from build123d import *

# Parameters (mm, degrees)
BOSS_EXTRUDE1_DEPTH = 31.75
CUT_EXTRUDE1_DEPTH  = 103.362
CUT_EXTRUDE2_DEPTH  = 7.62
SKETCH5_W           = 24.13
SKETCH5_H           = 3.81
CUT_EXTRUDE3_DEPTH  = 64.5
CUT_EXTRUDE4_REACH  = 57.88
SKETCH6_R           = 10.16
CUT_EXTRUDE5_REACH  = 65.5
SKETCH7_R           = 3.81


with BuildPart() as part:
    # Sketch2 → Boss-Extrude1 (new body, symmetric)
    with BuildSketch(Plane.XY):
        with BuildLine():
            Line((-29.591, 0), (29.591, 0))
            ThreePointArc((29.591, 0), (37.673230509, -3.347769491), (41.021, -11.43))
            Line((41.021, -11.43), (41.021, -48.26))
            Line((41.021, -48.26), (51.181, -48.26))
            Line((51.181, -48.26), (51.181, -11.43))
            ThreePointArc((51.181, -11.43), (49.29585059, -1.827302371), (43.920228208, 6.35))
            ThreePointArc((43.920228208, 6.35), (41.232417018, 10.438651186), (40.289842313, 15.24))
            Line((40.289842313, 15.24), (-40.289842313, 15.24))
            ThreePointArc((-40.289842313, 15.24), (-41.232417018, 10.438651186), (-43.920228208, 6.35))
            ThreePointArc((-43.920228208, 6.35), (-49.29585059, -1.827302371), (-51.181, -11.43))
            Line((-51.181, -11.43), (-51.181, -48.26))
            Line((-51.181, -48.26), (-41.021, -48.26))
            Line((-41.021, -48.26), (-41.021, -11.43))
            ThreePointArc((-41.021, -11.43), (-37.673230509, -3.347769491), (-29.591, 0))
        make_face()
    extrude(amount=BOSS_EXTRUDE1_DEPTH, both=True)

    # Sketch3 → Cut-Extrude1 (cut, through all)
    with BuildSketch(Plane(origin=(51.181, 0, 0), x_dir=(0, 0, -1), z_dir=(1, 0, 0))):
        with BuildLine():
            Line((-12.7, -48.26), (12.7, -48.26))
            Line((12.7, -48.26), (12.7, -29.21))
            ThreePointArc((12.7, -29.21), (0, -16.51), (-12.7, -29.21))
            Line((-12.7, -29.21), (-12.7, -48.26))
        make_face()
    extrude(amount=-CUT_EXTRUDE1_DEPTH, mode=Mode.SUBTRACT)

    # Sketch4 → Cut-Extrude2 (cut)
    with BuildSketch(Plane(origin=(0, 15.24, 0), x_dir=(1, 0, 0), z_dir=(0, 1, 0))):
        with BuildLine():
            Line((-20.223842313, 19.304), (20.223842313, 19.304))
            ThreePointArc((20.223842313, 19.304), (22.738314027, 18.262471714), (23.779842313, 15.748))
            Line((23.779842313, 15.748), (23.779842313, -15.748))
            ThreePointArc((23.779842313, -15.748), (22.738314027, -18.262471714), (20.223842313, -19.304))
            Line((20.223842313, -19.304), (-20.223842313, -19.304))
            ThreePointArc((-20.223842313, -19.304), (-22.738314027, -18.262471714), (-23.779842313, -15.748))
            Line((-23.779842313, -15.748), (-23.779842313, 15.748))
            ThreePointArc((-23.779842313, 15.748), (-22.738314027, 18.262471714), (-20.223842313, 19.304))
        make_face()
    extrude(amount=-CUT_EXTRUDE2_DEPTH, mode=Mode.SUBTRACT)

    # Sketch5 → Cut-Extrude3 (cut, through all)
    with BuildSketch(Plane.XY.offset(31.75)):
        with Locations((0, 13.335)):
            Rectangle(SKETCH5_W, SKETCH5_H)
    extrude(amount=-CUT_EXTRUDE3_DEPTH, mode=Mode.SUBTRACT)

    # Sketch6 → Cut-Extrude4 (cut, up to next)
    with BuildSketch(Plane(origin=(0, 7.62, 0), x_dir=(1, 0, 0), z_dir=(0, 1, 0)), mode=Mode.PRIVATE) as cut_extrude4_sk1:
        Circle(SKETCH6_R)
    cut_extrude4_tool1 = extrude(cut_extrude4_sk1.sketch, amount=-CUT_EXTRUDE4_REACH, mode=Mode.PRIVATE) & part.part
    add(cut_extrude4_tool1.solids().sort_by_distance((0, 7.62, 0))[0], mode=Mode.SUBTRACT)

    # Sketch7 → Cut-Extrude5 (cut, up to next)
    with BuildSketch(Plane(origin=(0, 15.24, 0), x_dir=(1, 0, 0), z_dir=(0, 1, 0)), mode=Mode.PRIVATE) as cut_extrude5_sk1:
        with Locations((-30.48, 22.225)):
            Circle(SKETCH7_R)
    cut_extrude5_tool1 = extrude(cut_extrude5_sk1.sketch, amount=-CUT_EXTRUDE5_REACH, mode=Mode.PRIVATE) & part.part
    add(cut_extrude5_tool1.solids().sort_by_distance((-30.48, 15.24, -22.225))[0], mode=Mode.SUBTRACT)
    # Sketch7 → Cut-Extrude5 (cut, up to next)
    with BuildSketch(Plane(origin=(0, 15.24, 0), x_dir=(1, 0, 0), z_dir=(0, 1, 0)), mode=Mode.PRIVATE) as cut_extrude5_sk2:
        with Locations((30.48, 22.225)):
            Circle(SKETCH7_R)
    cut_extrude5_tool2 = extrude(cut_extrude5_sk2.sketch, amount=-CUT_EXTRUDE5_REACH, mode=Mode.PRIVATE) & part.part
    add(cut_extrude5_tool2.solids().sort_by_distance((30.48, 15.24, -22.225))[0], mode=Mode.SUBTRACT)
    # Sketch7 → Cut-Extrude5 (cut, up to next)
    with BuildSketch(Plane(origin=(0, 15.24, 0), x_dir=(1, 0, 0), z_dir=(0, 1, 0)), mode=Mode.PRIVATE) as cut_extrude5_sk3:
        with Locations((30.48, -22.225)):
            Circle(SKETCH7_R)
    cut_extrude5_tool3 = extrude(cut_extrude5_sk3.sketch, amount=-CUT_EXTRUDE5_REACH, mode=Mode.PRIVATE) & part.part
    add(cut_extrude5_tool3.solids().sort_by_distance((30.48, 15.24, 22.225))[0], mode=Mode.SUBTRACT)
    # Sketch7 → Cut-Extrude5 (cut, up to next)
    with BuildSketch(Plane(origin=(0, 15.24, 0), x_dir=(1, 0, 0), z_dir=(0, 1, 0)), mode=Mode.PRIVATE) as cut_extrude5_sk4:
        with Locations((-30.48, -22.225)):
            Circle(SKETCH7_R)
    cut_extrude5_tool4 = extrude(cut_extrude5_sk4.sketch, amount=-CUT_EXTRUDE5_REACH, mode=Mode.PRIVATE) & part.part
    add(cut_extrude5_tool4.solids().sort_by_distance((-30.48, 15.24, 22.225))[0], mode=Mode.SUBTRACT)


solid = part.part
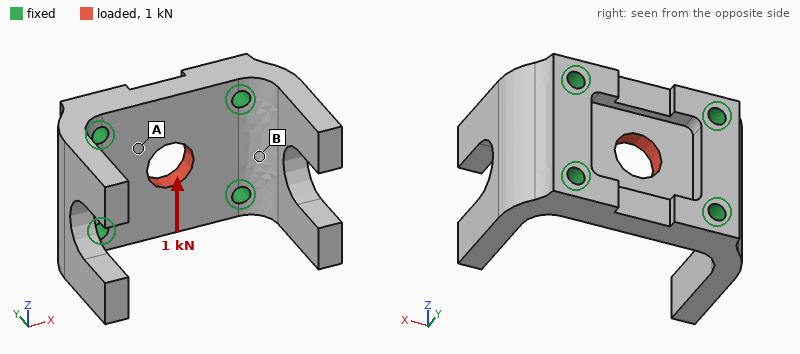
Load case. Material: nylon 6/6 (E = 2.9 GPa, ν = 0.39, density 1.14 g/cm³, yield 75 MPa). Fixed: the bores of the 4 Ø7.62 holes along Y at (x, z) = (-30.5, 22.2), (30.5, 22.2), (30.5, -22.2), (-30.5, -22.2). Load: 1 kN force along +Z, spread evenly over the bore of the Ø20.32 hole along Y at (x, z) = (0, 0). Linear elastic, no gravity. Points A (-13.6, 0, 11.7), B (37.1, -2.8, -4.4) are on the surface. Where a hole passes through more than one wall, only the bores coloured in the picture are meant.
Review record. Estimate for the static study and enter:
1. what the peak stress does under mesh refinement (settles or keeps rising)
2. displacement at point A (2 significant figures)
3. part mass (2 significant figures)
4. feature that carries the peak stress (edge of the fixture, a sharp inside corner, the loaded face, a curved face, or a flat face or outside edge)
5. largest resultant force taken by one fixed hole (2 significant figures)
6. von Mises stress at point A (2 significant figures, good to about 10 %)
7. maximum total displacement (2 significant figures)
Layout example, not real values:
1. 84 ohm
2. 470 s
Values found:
1. keeps rising
2. 16 µm
3. 130 g
4. edge of the fixture
5. 290 N
6. 1.9 MPa
7. 30 µm
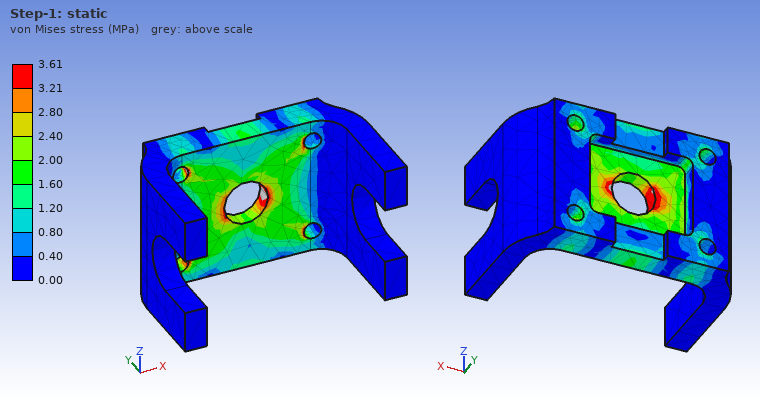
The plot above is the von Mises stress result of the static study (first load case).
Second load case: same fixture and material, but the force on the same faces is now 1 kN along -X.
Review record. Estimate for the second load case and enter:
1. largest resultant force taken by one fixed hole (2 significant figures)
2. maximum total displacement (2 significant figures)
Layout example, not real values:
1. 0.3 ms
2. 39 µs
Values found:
1. 260 N
2. 17 µm
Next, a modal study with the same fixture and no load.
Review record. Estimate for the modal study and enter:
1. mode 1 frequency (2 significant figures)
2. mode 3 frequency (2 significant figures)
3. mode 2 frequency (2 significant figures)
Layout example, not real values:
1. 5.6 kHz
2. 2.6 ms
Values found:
1. 1000 Hz
2. 1200 Hz
3. 1000 Hz
